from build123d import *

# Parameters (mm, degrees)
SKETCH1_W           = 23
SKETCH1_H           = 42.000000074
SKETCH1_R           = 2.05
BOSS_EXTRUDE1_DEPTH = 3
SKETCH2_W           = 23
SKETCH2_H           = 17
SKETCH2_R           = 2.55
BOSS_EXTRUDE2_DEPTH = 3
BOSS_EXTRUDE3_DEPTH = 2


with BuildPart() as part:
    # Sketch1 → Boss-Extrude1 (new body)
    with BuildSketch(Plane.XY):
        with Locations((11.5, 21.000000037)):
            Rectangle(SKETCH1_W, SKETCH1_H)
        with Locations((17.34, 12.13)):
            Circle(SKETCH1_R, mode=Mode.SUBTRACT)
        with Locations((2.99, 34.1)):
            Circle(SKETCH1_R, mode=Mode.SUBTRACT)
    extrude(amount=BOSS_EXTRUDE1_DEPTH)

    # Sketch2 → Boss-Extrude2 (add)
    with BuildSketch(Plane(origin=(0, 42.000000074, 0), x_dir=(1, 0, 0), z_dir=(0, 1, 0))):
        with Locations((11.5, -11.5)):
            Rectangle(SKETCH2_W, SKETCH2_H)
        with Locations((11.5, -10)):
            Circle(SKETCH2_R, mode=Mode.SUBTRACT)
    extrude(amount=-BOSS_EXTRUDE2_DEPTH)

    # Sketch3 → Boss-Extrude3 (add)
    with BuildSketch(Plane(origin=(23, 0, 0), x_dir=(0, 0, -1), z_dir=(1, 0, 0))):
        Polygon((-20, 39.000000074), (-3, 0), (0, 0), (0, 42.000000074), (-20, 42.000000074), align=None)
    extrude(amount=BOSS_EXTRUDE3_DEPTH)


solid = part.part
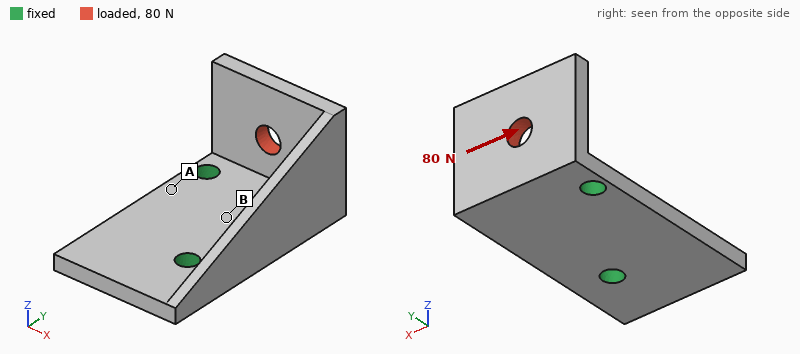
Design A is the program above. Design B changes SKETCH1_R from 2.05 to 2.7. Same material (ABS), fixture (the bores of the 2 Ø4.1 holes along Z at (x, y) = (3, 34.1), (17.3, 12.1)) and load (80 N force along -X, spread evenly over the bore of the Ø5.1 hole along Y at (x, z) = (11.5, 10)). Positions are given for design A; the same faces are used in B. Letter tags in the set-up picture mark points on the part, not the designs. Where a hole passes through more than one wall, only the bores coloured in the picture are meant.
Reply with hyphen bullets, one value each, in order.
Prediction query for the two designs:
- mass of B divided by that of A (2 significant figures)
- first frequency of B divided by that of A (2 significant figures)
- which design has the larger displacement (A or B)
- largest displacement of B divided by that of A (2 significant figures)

- 0.99
- 1.1
- A
- 0.81
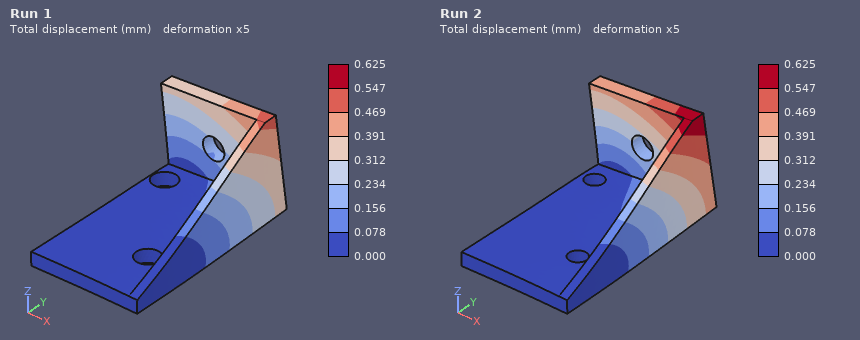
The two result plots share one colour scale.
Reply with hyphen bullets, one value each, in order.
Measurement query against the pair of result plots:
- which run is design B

- Run 1
